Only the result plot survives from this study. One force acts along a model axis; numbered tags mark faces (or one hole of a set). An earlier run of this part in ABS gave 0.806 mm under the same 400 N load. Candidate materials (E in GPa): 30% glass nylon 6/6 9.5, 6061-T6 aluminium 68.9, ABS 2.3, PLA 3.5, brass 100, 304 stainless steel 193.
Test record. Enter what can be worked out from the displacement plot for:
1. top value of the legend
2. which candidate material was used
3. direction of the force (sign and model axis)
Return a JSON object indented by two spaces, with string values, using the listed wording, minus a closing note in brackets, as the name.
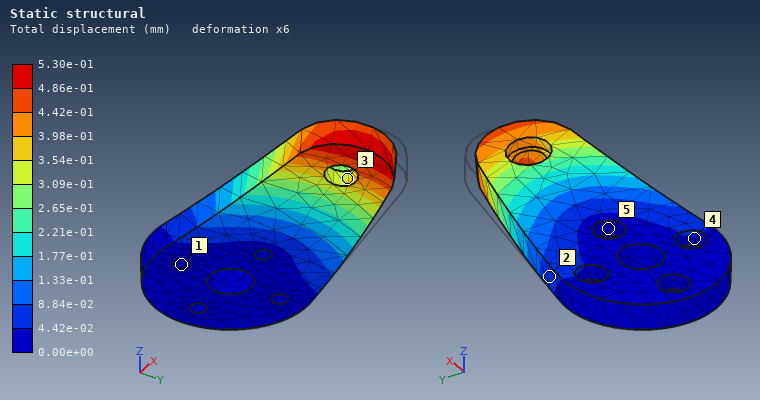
{
  "top value of the legend": "5.30e-01 mm",
  "which candidate material was used": "PLA",
  "direction of the force": "-Y"
}
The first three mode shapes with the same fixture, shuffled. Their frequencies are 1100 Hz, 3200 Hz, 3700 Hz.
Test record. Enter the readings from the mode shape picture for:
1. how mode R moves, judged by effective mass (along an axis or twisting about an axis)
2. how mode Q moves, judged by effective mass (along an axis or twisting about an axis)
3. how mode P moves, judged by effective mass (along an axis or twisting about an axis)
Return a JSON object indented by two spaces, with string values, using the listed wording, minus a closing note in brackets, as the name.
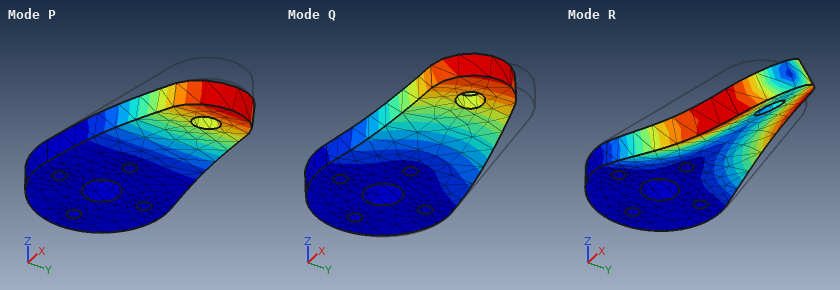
{
  "how mode R moves, judged by effective mass": "twisting about X",
  "how mode Q moves, judged by effective mass": "along Y",
  "how mode P moves, judged by effective mass": "along Z"
}
